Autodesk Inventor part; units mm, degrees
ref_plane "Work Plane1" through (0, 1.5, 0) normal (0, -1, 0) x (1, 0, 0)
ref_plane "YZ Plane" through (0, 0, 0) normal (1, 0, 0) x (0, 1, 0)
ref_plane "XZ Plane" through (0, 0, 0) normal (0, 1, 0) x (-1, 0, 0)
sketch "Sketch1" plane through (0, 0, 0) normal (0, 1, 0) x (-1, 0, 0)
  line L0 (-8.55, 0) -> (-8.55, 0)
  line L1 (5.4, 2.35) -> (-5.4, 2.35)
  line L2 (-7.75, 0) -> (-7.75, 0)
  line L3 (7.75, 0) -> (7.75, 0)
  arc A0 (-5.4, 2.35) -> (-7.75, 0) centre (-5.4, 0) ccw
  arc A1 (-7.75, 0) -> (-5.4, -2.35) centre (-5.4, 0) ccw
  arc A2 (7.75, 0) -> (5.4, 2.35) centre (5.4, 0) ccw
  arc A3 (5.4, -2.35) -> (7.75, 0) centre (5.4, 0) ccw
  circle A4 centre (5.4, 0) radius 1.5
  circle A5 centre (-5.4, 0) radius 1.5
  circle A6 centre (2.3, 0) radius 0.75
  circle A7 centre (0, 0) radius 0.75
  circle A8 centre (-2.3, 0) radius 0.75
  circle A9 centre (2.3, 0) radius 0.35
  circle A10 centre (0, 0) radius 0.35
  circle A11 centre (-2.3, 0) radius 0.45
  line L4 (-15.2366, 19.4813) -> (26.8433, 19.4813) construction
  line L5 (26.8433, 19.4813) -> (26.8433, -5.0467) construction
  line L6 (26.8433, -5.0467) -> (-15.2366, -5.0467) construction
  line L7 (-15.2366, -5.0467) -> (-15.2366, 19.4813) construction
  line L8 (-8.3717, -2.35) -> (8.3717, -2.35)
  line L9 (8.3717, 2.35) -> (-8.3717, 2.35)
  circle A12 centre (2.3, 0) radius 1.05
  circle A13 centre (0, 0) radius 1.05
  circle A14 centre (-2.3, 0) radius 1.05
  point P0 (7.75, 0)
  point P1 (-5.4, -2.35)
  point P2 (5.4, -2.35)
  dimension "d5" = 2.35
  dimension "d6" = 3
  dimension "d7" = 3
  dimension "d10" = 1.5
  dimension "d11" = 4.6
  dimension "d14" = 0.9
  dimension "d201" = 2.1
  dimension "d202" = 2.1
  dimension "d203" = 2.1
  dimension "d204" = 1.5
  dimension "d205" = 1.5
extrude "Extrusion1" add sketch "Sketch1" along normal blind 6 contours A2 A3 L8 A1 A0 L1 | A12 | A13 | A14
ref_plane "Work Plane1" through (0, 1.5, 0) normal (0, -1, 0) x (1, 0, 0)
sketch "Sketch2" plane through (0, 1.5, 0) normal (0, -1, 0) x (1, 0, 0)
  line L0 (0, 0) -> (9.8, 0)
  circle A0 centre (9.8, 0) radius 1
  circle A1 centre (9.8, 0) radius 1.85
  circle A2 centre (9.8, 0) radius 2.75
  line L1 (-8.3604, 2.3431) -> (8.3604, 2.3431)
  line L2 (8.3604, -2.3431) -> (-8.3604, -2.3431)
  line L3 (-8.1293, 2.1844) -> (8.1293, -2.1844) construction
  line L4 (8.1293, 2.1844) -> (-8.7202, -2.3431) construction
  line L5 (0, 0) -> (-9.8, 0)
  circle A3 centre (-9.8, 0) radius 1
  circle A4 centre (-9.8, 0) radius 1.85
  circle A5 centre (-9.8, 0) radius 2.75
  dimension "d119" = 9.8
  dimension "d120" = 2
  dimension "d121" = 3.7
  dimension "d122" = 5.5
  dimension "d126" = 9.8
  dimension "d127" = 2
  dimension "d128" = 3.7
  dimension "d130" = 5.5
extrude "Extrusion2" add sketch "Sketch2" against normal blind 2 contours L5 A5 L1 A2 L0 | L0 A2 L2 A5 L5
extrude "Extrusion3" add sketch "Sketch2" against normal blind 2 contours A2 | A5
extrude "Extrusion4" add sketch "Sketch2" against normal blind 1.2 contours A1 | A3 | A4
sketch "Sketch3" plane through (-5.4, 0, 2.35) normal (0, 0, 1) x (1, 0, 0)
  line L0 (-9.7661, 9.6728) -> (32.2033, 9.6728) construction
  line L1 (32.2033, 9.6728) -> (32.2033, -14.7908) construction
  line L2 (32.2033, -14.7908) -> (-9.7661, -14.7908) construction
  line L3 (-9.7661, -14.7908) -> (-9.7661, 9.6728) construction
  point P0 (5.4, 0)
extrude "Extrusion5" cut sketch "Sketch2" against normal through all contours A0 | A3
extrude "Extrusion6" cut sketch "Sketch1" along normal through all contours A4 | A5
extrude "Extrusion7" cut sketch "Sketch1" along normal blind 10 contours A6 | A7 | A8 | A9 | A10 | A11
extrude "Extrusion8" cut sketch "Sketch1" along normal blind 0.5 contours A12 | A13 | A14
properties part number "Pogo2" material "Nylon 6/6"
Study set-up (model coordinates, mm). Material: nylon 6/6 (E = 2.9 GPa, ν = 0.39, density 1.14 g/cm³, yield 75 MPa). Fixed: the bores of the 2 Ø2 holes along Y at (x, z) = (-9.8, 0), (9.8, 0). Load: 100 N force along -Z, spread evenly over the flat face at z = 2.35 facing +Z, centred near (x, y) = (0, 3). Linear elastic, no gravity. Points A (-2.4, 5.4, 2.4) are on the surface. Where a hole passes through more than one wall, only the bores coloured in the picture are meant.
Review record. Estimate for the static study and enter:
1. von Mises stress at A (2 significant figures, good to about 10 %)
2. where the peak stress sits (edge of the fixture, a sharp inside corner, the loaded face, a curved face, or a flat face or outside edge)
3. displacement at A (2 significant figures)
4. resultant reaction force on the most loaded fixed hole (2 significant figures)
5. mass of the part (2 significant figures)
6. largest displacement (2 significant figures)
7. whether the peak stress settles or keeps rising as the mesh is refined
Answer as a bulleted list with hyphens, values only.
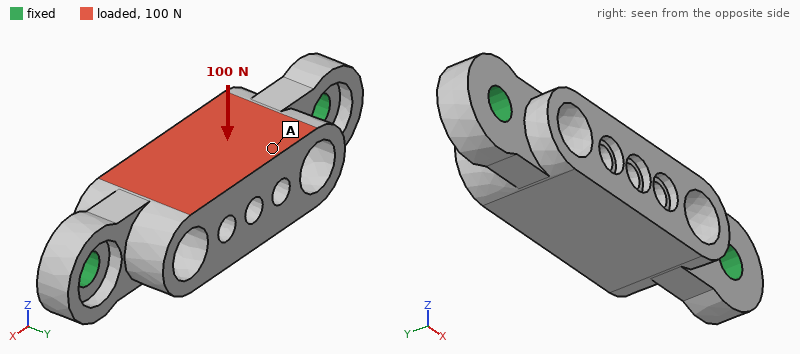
- 10.0 MPa
- edge of the fixture
- 0.16 mm
- 50 N
- 0.41 g
- 0.18 mm
- keeps rising
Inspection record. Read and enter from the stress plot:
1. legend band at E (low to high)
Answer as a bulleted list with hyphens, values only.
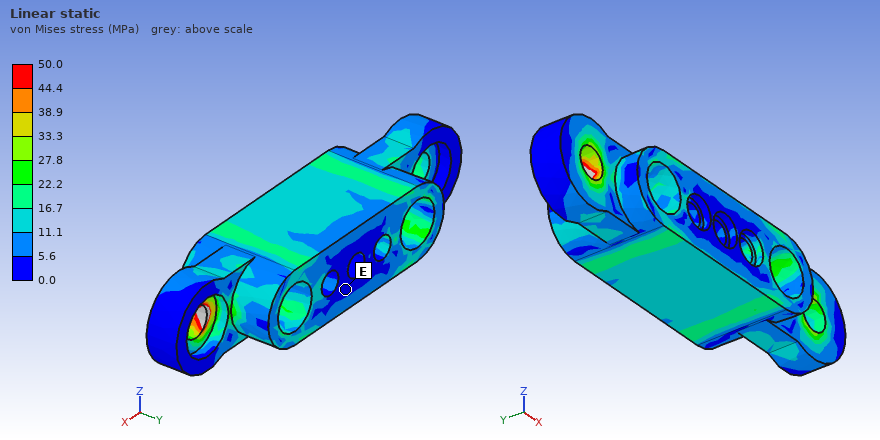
- 0.0 to 5.6 MPa
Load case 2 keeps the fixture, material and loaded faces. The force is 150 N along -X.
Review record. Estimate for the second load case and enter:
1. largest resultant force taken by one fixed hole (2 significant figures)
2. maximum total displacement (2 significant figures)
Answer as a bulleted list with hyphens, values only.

- 78 N
- 38 µm
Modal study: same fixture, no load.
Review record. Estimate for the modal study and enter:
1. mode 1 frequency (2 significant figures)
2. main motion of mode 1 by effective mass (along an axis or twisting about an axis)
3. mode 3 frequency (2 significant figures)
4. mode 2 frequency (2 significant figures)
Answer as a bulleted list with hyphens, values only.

- 7500 Hz
- along Z
- 10000 Hz
- 10000 Hz
